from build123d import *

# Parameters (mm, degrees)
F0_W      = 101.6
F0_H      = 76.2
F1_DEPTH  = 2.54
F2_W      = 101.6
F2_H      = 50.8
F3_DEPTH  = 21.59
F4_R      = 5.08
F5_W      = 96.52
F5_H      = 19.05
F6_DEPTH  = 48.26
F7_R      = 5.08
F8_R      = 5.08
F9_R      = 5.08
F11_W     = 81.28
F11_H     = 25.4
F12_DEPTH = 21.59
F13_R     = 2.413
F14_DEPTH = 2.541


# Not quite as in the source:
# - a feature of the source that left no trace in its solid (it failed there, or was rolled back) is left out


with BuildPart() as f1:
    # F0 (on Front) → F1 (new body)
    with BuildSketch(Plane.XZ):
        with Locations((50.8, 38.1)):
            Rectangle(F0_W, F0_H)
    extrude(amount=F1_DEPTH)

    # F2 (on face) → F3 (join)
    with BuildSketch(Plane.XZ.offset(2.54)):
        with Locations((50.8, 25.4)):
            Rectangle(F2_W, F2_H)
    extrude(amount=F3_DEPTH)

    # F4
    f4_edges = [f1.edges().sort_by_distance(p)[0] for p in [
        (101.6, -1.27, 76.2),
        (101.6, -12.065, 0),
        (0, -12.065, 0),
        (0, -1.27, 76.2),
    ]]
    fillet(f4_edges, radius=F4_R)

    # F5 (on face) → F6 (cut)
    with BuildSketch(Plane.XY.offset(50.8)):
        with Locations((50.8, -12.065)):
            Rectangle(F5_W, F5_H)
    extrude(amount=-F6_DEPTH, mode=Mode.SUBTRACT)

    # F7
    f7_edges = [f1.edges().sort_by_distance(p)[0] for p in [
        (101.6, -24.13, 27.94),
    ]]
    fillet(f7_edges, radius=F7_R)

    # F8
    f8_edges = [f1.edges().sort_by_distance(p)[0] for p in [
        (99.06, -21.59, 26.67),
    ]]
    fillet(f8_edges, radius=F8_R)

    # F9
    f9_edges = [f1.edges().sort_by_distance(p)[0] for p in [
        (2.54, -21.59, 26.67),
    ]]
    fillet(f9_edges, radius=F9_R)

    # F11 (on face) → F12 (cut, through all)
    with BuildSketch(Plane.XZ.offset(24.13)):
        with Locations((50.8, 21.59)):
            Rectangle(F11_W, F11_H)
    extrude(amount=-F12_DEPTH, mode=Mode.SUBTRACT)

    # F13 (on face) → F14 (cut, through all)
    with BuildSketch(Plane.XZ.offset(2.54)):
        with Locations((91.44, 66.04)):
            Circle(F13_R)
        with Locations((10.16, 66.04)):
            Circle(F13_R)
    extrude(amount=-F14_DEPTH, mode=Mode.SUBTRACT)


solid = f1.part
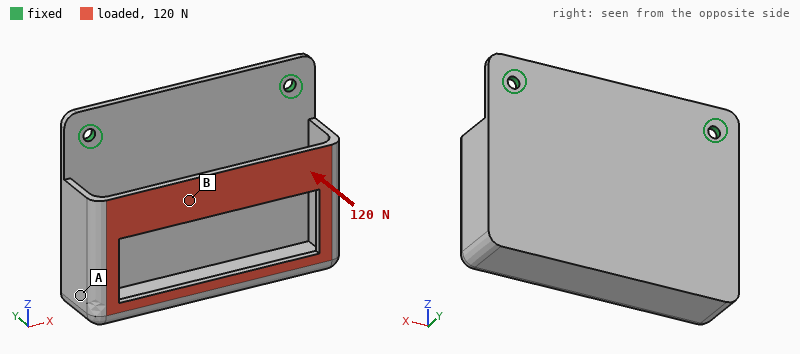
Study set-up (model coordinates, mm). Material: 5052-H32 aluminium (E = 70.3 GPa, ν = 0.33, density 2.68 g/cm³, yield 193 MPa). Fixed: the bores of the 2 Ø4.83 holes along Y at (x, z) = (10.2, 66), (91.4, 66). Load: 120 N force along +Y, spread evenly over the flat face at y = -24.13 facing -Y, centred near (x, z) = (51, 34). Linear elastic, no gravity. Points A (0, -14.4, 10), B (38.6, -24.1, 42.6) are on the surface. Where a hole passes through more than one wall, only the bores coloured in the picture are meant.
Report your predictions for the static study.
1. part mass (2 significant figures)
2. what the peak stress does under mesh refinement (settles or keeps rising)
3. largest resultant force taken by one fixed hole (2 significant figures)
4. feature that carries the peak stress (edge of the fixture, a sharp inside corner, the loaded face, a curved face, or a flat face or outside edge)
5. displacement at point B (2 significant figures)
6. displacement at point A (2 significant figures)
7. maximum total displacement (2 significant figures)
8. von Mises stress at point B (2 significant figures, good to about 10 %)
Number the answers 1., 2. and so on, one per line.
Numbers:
1. 97 g
2. keeps rising
3. 61 N
4. edge of the fixture
5. 0.31 mm
6. 0.40 mm
7. 0.49 mm
8. 17 MPa
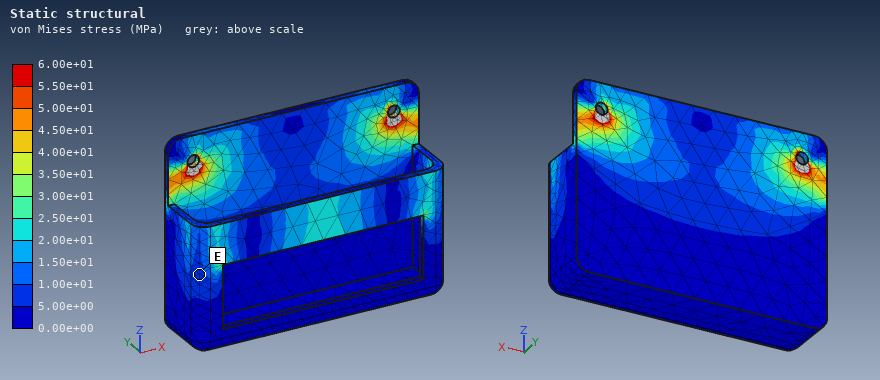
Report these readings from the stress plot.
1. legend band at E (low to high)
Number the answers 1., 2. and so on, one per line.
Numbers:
1. 5.00e+00 to 1.00e+01 MPa
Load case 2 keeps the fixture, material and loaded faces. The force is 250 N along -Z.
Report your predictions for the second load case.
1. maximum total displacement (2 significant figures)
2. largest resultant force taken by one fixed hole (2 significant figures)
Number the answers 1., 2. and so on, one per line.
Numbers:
1. 1.1 mm
2. 130 N
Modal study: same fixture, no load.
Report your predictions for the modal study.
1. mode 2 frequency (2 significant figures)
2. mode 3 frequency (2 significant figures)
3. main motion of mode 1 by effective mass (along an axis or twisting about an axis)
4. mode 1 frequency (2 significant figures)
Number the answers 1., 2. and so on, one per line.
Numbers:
1. 740 Hz
2. 1300 Hz
3. along Y
4. 250 Hz
